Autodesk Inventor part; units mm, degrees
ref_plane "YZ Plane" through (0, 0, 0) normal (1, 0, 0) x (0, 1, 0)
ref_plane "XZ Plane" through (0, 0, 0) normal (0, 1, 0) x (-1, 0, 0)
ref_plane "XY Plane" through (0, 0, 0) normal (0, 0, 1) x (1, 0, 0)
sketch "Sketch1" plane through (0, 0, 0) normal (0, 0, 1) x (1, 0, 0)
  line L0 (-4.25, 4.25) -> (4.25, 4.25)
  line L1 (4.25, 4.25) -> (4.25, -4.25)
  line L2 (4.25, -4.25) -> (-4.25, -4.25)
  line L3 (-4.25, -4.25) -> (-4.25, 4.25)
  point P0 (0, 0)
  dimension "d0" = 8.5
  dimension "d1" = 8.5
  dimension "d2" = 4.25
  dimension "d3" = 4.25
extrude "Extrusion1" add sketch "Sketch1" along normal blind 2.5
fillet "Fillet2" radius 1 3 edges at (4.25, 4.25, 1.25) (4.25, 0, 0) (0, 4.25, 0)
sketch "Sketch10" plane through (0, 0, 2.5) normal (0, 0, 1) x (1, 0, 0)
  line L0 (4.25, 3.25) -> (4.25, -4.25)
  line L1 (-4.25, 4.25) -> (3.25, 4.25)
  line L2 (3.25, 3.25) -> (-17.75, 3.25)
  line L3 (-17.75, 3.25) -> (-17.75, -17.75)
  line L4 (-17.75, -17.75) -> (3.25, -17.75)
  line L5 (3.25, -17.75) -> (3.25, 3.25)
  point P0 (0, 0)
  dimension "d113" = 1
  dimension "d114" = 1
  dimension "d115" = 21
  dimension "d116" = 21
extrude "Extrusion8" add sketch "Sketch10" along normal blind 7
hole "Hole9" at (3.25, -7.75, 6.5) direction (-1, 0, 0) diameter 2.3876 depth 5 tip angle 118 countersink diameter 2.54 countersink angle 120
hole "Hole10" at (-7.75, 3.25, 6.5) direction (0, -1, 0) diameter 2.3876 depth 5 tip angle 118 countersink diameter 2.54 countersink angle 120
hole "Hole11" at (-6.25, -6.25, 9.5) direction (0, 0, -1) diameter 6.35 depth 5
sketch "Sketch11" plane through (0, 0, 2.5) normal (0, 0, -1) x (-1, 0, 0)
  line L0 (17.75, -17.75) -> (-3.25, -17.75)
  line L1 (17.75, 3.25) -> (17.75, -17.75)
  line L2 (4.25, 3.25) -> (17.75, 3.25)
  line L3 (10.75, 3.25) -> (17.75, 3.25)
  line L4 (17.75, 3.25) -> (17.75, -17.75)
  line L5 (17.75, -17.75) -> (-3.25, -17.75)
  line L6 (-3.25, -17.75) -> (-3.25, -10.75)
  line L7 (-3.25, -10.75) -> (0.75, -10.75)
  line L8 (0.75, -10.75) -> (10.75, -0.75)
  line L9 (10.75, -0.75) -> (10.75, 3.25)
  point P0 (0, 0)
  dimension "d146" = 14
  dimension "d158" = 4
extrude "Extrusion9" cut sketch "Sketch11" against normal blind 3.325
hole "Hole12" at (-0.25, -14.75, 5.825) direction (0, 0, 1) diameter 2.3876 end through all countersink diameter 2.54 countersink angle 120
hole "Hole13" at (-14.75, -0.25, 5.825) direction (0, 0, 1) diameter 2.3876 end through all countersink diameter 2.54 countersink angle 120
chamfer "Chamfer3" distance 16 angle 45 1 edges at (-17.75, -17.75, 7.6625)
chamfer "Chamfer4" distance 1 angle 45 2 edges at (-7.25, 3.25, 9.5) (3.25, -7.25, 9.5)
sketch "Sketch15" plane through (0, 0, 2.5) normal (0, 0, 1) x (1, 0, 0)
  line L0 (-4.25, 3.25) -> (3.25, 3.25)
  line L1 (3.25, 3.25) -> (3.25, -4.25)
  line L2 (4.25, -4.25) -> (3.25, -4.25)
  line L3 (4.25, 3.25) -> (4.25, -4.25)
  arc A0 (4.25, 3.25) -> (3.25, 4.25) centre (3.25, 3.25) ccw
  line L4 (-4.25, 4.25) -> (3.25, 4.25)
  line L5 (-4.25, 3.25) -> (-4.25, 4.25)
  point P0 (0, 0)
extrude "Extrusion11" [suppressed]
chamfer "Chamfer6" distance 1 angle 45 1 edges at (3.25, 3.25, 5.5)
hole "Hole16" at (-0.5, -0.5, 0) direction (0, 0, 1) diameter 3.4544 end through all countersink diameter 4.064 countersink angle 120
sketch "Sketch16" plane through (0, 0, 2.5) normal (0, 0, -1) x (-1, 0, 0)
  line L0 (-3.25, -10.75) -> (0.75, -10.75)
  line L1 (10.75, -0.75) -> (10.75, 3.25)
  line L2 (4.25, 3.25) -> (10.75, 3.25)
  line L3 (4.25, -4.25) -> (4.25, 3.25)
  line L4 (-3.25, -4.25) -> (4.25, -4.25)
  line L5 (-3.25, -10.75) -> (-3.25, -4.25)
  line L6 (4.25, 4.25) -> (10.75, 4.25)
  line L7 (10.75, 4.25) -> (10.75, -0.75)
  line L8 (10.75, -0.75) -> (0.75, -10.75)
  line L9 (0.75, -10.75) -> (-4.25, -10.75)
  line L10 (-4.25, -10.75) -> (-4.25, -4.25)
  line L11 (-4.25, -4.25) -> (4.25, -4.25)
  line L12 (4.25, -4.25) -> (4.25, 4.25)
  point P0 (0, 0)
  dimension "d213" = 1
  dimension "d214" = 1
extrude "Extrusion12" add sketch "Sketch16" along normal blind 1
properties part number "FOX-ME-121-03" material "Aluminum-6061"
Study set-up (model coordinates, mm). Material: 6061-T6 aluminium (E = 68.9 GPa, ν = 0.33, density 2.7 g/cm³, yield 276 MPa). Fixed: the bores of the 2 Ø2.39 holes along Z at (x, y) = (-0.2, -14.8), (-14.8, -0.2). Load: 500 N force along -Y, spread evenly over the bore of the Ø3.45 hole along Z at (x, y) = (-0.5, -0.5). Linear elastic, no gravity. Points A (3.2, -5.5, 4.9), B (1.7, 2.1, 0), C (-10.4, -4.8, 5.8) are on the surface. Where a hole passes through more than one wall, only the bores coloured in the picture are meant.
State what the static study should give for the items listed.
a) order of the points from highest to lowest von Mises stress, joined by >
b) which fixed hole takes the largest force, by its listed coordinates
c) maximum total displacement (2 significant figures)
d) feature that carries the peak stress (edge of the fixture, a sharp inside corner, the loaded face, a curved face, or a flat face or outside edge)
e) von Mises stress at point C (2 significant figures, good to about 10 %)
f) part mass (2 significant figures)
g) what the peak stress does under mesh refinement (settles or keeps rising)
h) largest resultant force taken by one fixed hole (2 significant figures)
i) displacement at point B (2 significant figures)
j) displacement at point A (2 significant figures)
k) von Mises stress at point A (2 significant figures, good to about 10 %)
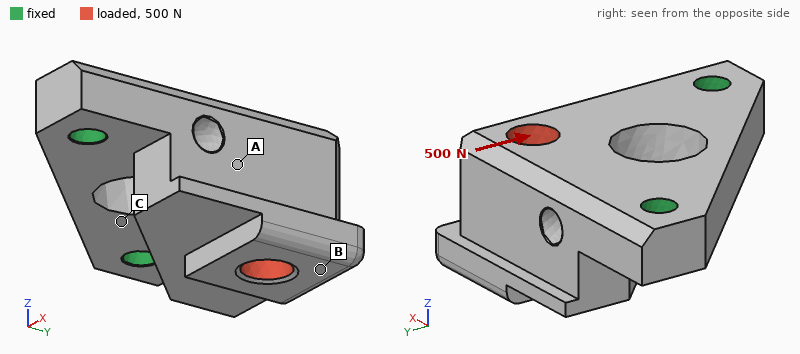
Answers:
A > C > B
(-0.2, -14.8)
23 µm
edge of the fixture
9.9 MPa
4.3 g
keeps rising
420 N
20 µm
11 µm
18 MPa
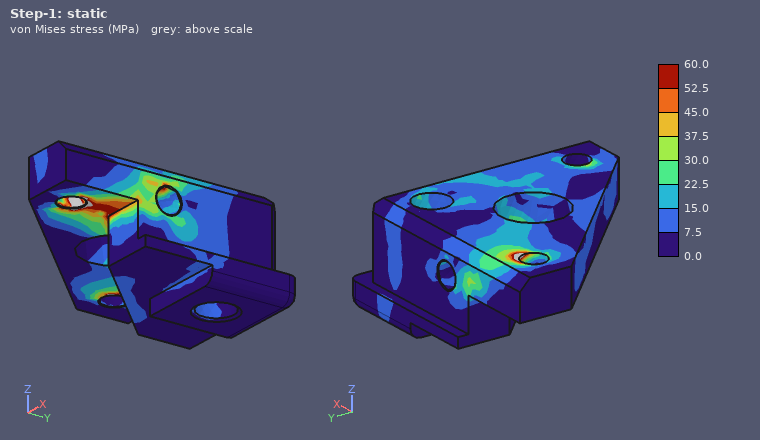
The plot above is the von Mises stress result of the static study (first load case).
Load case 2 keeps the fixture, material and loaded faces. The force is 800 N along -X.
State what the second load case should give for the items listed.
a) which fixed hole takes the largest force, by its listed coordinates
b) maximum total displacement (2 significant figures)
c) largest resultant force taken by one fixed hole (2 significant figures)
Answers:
(-14.8, -0.2)
37 µm
680 N
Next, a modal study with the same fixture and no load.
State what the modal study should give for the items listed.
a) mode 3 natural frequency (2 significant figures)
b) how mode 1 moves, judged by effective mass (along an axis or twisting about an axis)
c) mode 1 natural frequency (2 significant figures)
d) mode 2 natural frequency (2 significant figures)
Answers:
37 kHz
along Z
10 kHz
36 kHz
